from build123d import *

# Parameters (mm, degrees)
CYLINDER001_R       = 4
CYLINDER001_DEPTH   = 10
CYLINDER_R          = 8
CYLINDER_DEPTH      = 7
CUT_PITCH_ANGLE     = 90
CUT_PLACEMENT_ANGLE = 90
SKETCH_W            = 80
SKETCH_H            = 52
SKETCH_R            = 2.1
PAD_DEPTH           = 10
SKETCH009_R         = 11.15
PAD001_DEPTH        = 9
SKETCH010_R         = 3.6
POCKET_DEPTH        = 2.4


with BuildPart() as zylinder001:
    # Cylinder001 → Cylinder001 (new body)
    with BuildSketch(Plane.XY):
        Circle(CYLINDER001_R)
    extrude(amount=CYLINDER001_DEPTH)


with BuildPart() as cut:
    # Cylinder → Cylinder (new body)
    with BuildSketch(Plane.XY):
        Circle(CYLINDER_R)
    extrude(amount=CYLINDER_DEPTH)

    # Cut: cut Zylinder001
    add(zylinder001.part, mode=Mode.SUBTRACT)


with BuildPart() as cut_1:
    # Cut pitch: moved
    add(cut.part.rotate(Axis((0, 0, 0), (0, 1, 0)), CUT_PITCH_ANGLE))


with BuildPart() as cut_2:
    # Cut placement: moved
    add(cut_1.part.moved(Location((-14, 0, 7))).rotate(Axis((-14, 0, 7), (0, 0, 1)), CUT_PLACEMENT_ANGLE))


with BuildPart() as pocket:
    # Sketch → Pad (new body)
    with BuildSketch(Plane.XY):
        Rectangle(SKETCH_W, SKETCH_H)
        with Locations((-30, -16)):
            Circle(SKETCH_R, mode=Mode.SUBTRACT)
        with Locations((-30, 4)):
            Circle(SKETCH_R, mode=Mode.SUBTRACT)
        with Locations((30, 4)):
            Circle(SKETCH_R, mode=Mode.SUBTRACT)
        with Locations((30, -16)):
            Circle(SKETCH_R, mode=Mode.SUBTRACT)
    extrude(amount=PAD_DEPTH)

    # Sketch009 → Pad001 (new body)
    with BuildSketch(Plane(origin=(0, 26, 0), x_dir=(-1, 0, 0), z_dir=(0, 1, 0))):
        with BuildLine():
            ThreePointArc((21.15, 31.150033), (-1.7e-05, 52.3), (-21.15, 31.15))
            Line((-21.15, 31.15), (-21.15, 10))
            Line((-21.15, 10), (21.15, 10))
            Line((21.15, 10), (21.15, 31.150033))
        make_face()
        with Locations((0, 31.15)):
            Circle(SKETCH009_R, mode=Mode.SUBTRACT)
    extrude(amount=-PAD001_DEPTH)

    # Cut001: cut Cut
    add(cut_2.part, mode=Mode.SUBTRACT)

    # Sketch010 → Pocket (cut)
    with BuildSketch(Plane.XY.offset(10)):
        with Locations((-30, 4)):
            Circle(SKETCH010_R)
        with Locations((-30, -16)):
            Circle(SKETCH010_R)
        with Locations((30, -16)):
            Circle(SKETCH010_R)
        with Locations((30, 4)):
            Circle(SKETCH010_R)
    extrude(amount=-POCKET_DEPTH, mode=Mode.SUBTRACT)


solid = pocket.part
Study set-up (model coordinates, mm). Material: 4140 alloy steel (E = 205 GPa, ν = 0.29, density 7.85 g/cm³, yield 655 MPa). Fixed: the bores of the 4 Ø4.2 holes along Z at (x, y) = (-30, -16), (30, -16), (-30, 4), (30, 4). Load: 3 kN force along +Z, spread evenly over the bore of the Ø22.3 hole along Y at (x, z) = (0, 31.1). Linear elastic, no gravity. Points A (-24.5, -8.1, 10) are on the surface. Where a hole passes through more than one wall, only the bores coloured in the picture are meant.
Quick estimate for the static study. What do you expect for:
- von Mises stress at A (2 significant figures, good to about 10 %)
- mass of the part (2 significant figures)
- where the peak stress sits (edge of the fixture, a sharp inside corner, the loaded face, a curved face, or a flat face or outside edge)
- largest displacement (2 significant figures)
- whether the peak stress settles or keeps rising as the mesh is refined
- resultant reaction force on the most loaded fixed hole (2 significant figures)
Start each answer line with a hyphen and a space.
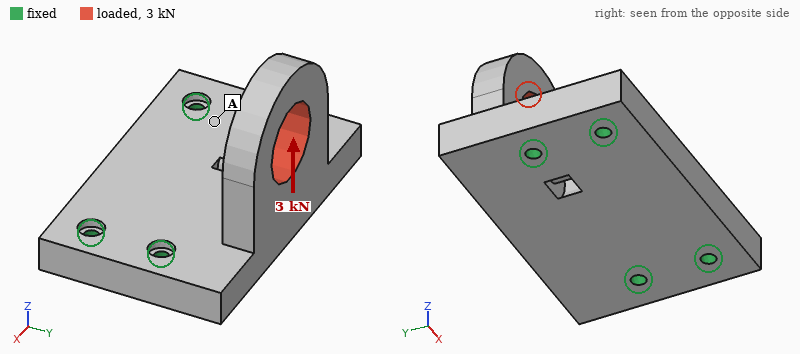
- 16 MPa
- 400 g
- edge of the fixture
- 41 µm
- keeps rising
- 2.3 kN
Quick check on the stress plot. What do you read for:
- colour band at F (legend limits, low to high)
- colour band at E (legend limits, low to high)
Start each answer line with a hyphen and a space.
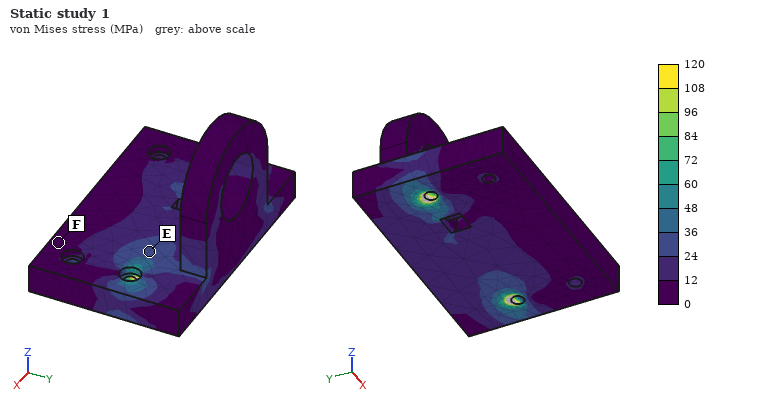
- 0 to 12 MPa
- 24 to 36 MPa
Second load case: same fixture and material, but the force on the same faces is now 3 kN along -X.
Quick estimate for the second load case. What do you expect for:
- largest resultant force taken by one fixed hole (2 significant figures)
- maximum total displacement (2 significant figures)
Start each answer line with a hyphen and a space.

- 2.3 kN
- 30 µm
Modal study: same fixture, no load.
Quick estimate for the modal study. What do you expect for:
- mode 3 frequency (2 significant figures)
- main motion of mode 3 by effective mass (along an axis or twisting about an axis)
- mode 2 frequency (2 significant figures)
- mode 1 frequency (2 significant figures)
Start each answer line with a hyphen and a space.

- 6700 Hz
- along Z
- 6200 Hz
- 2900 Hz
